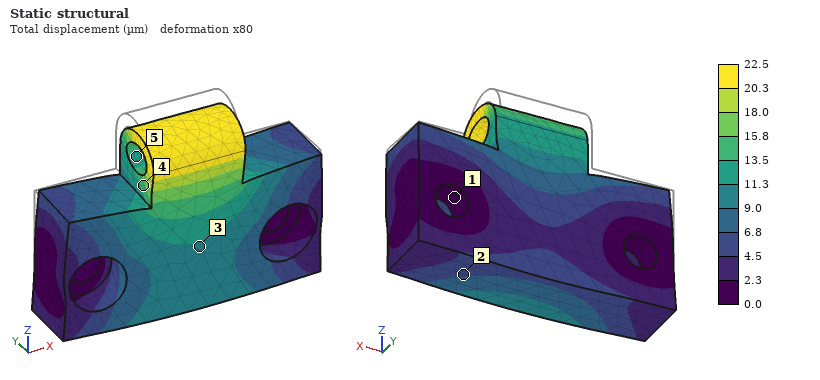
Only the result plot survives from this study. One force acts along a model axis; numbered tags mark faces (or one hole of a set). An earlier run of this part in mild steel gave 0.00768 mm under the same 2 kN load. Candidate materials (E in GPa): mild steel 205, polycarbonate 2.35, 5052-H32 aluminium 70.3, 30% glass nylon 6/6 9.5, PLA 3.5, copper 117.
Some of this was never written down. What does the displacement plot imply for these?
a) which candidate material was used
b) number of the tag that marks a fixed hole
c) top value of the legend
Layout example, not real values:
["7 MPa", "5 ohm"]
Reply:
["5052-H32 aluminium", "1", "22.5 µm"]
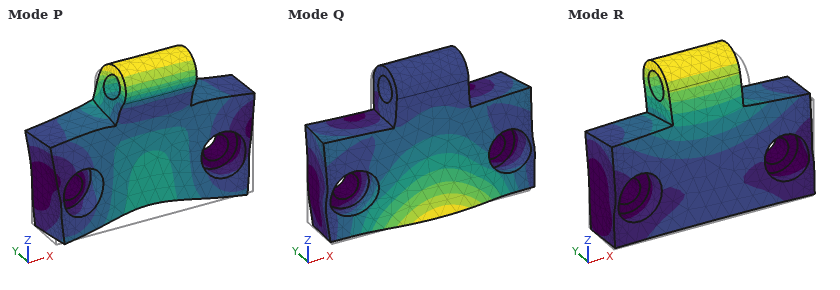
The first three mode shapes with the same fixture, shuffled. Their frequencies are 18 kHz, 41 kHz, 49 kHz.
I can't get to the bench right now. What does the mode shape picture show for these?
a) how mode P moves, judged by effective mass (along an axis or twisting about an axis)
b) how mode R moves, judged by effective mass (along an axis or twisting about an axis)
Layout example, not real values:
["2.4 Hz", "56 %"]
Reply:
["along Z", "along Y"]
